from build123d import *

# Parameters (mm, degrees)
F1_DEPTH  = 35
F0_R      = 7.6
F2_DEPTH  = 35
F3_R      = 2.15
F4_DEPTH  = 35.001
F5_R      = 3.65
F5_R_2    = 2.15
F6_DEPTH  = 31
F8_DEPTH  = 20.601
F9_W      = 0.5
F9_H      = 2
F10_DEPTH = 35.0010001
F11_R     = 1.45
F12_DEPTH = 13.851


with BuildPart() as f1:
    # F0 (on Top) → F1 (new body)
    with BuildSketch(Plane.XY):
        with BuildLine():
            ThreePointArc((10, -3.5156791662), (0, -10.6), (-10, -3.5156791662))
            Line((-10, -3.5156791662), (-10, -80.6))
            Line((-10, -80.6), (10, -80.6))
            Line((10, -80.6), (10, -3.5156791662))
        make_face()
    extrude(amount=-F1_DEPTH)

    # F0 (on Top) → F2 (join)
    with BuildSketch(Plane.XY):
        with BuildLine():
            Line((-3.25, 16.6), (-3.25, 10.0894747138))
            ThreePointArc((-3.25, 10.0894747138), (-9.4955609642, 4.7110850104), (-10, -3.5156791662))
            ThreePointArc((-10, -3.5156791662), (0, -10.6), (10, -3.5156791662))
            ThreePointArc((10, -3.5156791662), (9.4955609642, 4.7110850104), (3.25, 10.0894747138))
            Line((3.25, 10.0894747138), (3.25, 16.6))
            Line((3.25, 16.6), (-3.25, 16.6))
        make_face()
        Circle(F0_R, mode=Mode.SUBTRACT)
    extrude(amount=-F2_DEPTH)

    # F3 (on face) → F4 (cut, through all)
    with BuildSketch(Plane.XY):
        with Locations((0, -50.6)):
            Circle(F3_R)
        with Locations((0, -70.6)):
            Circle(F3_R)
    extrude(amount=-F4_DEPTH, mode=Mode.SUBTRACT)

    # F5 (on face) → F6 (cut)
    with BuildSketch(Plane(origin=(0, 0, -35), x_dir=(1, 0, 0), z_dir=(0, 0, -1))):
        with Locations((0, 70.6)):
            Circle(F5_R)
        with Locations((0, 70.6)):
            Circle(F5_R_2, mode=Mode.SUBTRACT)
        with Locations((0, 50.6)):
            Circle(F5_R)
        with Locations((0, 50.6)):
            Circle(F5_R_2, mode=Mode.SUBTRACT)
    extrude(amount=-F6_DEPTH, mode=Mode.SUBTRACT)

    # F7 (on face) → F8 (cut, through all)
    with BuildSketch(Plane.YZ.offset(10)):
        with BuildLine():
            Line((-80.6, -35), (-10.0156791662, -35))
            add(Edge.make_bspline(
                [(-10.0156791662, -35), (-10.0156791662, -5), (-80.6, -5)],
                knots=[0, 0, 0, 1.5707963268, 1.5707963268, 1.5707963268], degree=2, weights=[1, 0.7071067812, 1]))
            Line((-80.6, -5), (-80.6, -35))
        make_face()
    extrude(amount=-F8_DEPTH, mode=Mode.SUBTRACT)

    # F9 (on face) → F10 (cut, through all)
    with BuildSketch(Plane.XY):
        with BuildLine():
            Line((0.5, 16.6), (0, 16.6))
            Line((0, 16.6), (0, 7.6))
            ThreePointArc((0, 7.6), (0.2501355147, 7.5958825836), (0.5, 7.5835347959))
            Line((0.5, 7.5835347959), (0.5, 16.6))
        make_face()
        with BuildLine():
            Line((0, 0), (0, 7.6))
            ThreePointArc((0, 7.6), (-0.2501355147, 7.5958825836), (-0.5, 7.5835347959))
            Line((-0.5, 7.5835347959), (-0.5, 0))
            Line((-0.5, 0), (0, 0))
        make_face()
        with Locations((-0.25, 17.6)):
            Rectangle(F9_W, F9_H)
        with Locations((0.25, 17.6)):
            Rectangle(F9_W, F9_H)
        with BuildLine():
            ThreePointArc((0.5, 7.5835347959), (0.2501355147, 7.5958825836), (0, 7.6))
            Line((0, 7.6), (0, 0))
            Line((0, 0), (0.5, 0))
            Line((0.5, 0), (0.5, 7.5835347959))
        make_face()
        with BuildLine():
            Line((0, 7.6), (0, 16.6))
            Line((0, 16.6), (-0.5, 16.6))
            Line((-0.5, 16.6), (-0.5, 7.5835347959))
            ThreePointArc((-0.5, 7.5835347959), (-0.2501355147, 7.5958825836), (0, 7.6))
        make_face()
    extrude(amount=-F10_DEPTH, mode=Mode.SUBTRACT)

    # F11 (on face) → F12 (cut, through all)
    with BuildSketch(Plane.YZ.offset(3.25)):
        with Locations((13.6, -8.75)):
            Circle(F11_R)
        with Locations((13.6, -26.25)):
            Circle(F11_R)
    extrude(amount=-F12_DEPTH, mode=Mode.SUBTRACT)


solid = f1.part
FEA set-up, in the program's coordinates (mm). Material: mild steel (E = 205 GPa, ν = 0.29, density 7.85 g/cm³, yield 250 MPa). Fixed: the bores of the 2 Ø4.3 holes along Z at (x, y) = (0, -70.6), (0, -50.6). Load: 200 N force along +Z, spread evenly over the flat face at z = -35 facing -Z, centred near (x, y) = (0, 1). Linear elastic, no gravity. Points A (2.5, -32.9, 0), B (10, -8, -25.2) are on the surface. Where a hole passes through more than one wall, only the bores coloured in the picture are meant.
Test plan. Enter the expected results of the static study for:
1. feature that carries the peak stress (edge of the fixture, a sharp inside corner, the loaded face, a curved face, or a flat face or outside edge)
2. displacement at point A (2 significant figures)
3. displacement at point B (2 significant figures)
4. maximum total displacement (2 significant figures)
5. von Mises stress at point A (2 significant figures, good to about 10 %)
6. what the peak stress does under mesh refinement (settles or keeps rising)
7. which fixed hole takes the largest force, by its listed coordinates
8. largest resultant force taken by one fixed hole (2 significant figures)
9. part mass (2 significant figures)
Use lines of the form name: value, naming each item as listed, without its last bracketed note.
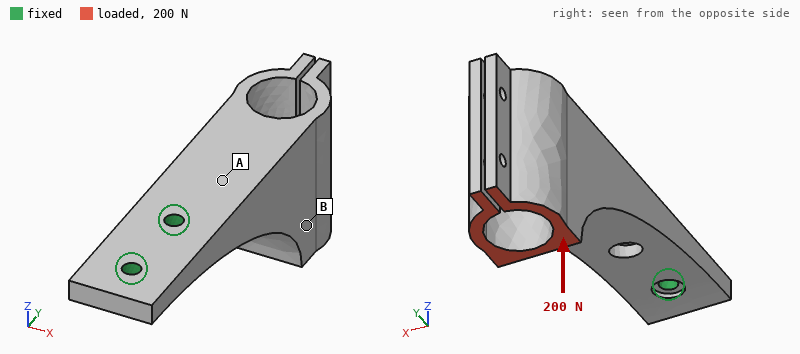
feature that carries the peak stress: edge of the fixture
displacement at point A: 13 µm
displacement at point B: 43 µm
maximum total displacement: 70 µm
von Mises stress at point A: 14 MPa
what the peak stress does under mesh refinement: keeps rising
which fixed hole takes the largest force, by its listed coordinates: (0, -50.6)
largest resultant force taken by one fixed hole: 700 N
part mass: 190 g
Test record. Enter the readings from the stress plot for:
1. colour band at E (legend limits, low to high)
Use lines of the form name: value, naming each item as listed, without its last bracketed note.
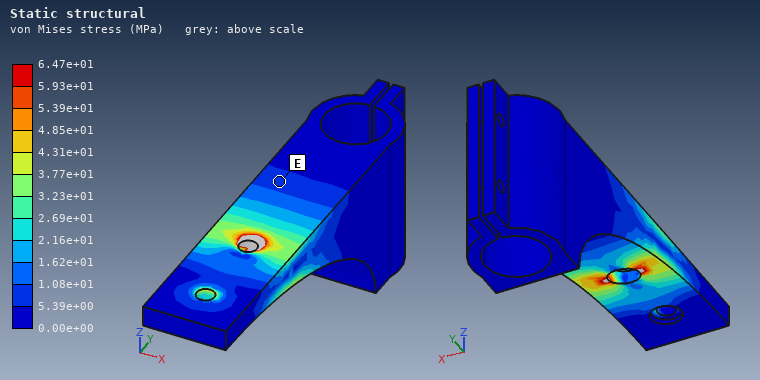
colour band at E: 5.39e+00 to 1.08e+01 MPa
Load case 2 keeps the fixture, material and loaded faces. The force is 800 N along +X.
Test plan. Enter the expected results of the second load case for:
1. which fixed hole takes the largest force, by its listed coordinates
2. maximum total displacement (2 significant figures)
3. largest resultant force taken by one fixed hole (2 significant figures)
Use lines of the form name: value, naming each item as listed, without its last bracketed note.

which fixed hole takes the largest force, by its listed coordinates: (0, -50.6)
maximum total displacement: 0.20 mm
largest resultant force taken by one fixed hole: 2.3 kN
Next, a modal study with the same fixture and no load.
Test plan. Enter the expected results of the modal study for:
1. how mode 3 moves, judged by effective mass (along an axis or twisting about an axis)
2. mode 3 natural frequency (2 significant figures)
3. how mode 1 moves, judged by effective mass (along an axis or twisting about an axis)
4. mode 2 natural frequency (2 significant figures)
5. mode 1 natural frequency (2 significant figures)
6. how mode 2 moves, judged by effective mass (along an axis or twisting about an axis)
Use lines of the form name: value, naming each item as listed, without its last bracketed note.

how mode 3 moves, judged by effective mass: twisting about Y
mode 3 natural frequency: 3900 Hz
how mode 1 moves, judged by effective mass: along Z
mode 2 natural frequency: 1800 Hz
mode 1 natural frequency: 1100 Hz
how mode 2 moves, judged by effective mass: along X
